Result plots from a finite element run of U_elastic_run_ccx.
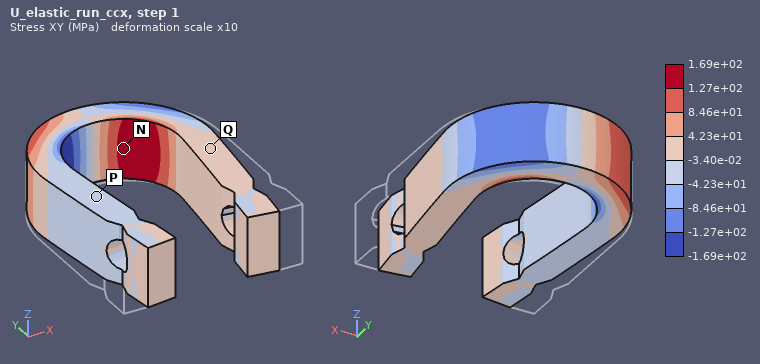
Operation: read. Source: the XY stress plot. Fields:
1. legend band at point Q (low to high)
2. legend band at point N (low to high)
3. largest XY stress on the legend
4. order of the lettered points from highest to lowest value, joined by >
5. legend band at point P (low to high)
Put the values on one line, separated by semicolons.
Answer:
-3.40e-02 to 4.23e+01 MPa; 1.27e+02 to 1.69e+02 MPa; 1.69e+02 MPa; N > Q > P; -4.23e+01 to -3.40e-02 MPa
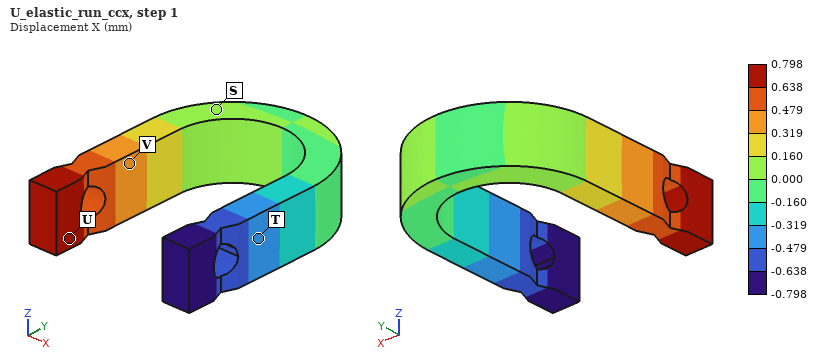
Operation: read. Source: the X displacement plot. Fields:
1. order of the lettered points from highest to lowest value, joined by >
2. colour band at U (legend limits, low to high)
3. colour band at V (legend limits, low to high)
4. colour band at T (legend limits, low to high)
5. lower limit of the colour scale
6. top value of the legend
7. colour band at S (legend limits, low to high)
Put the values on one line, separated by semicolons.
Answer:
U > V > S > T; 0.638 to 0.798 mm; 0.319 to 0.479 mm; -0.479 to -0.319 mm; -0.798 mm; 0.798 mm; 0.000 to 0.160 mm
